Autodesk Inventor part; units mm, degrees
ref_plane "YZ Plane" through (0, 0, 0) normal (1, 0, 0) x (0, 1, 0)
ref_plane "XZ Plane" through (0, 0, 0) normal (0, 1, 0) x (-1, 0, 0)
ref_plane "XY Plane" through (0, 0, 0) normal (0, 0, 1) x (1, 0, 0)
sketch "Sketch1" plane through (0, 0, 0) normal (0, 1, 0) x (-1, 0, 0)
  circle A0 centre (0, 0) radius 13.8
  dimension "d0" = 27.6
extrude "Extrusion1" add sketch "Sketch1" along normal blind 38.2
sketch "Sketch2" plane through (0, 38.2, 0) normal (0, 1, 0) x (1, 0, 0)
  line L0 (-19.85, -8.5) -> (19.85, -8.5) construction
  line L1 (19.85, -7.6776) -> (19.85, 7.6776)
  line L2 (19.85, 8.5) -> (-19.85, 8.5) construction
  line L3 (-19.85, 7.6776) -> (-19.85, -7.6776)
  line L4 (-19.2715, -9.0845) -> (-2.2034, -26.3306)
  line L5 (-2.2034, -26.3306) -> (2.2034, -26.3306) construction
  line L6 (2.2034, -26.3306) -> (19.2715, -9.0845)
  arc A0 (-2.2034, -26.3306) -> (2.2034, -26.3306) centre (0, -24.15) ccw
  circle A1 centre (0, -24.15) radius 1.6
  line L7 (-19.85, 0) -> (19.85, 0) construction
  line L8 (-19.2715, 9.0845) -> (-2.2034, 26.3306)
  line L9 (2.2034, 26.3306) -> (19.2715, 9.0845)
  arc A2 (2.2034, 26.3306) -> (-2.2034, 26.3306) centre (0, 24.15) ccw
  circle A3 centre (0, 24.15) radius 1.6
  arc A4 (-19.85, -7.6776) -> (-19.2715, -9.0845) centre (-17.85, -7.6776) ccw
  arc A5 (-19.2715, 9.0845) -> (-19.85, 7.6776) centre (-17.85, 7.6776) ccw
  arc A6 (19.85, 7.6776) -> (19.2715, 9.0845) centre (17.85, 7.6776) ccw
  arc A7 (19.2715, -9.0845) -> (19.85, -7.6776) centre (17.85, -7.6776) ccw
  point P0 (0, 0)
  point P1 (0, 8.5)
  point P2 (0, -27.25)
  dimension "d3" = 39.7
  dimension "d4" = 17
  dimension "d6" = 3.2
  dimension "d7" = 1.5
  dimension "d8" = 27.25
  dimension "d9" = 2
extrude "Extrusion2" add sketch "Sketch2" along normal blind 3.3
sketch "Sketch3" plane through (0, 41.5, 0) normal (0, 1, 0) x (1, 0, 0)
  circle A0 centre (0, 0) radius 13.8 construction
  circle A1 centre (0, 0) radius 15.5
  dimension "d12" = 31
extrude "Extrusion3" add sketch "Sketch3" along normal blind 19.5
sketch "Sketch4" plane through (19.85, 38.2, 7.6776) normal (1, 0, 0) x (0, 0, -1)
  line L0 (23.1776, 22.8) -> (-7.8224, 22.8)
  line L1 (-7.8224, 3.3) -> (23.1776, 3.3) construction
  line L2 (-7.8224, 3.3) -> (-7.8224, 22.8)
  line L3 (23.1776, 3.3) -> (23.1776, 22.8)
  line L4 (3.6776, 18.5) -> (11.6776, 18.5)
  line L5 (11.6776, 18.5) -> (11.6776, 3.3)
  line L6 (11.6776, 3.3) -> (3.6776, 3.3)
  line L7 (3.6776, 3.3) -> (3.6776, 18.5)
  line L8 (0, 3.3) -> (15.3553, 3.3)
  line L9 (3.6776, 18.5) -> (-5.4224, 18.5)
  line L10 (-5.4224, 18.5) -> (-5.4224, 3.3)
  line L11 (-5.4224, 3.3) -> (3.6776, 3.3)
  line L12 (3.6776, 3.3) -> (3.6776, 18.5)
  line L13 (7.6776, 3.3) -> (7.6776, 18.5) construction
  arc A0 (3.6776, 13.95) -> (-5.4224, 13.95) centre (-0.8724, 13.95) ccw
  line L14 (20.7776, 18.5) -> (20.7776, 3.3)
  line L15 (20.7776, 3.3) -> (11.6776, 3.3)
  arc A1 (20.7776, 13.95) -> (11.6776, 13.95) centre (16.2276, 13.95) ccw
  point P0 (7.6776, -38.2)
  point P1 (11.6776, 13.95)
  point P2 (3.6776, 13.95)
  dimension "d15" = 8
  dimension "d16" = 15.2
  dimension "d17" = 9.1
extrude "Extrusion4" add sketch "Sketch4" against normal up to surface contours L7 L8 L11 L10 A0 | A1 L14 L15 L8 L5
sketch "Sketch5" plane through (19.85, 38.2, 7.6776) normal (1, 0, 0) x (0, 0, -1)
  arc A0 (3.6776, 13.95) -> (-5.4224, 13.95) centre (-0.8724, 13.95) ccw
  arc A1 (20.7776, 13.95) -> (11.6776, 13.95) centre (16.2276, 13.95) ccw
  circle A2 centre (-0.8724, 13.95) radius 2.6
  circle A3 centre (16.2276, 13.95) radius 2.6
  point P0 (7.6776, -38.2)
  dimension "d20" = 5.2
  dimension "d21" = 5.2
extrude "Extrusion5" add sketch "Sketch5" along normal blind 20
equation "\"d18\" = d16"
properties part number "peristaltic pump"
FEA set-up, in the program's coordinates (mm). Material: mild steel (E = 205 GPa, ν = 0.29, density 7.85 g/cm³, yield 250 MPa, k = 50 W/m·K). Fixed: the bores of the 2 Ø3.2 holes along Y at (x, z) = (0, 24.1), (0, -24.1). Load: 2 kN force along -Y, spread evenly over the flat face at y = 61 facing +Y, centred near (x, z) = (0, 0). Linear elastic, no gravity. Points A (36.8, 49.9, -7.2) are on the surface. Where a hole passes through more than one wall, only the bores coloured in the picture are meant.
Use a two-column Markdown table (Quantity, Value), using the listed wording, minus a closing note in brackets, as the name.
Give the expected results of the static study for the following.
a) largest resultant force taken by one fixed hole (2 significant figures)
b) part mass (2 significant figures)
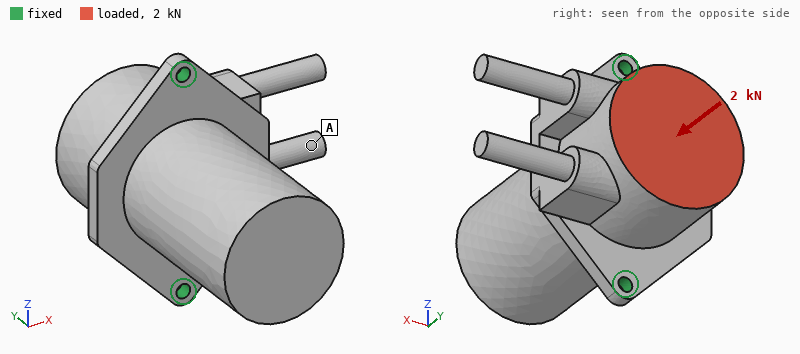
| Quantity | Value |
|---|---|
| largest resultant force taken by one fixed hole | 1.0 kN |
| part mass | 350 g |
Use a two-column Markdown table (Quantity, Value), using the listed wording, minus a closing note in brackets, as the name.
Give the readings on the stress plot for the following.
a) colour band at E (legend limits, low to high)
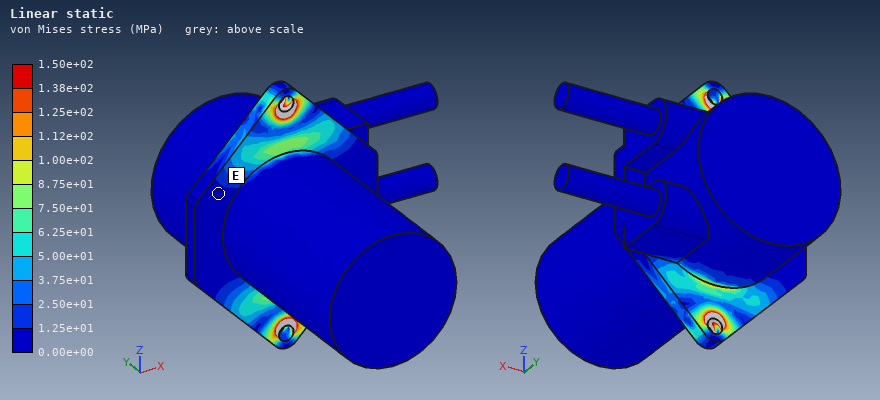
| Quantity | Value |
|---|---|
| colour band at E | 0.00e+00 to 1.25e+01 MPa |
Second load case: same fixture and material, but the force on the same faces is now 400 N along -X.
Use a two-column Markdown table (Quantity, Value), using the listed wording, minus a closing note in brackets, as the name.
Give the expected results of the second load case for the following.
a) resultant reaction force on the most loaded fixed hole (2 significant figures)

| Quantity | Value |
|---|---|
| resultant reaction force on the most loaded fixed hole | 200 N |
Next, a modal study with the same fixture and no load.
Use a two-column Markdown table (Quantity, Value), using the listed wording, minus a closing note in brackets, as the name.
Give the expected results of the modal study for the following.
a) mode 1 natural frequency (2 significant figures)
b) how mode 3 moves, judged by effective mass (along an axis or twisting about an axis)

| Quantity | Value |
|---|---|
| mode 1 natural frequency | 730 Hz |
| how mode 3 moves, judged by effective mass | along Y |
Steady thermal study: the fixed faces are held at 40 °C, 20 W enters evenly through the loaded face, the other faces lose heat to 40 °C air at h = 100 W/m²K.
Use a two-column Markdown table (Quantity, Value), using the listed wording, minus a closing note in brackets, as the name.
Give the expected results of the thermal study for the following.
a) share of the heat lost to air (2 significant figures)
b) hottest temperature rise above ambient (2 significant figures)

| Quantity | Value |
|---|---|
| share of the heat lost to air | 67 % |
| hottest temperature rise above ambient | 26 K |
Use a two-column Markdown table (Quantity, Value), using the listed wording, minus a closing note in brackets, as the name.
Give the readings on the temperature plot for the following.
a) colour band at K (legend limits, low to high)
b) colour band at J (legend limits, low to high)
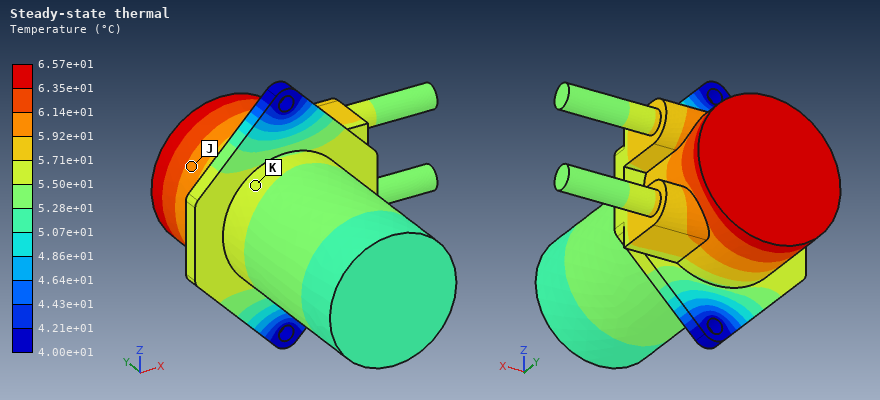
| Quantity | Value |
|---|---|
| colour band at K | 5.50e+01 to 5.71e+01 °C |
| colour band at J | 5.92e+01 to 6.14e+01 °C |
